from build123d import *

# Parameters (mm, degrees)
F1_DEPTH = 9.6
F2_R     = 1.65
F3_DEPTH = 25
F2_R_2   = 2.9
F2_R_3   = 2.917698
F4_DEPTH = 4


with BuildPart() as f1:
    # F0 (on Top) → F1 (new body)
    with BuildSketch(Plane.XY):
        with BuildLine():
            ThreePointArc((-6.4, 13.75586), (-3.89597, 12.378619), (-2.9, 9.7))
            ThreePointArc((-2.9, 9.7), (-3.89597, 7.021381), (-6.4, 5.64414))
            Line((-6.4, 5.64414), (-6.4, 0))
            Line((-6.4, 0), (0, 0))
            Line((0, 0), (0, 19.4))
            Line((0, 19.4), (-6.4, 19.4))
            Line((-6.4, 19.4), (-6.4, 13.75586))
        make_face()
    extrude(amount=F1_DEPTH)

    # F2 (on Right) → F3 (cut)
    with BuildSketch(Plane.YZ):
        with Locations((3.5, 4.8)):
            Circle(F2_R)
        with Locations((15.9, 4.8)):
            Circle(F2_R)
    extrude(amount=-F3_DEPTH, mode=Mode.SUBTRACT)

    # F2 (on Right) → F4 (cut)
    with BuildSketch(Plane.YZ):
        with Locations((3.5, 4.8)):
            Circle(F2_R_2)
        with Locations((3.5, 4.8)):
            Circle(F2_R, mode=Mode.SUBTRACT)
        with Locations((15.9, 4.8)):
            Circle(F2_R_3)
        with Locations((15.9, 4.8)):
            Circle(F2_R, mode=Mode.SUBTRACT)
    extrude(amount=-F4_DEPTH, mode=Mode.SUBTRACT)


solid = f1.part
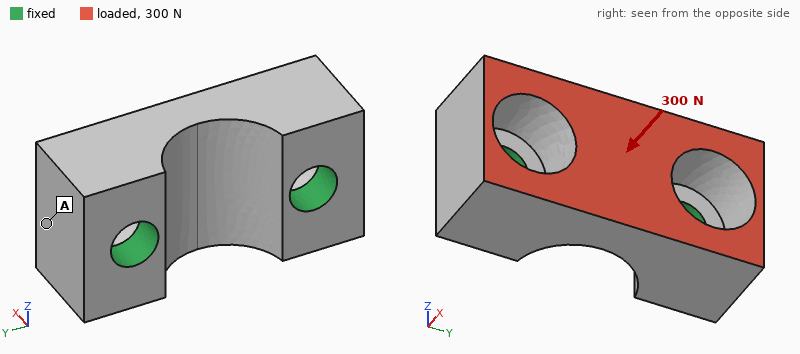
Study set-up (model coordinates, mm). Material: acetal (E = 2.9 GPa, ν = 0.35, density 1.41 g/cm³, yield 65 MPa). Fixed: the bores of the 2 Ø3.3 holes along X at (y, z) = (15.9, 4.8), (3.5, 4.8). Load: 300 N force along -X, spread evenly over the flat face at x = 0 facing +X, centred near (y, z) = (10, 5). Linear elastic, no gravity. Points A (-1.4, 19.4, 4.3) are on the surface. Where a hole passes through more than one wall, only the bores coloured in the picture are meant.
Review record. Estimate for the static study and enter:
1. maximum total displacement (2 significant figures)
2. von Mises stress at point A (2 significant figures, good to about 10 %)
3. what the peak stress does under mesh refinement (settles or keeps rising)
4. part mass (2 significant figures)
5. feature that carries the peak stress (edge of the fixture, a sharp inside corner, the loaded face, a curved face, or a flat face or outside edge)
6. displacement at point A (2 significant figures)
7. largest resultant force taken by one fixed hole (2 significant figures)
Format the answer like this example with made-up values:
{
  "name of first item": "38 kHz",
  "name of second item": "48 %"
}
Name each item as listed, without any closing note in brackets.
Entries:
{
  "maximum total displacement": "27 µm",
  "von Mises stress at point A": "4.2 MPa",
  "what the peak stress does under mesh refinement": "keeps rising",
  "part mass": "1.0 g",
  "feature that carries the peak stress": "a sharp inside corner",
  "displacement at point A": "8.4 µm",
  "largest resultant force taken by one fixed hole": "160 N"
}
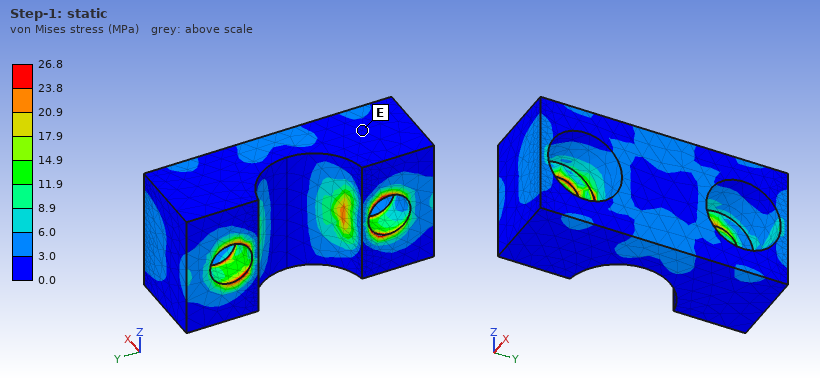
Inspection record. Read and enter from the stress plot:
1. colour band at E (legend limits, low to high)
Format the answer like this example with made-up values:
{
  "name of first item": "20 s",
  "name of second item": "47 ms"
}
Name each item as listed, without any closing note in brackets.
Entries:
{
  "colour band at E": "0.0 to 3.0 MPa"
}
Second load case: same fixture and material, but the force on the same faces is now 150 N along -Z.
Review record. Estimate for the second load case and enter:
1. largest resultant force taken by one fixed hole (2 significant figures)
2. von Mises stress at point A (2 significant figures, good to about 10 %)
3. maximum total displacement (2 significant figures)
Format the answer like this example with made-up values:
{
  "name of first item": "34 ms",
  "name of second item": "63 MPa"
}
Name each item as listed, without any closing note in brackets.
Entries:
{
  "largest resultant force taken by one fixed hole": "75 N",
  "von Mises stress at point A": "11 MPa",
  "maximum total displacement": "82 µm"
}
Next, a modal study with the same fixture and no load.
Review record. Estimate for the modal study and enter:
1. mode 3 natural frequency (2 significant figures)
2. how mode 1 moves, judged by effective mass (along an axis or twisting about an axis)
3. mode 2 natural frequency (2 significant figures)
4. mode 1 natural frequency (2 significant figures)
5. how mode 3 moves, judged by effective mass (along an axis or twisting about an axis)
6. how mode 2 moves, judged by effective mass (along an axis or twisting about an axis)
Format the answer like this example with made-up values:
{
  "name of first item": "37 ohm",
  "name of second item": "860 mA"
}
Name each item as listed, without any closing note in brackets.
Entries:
{
  "mode 3 natural frequency": "19 kHz",
  "how mode 1 moves, judged by effective mass": "along Z",
  "mode 2 natural frequency": "17 kHz",
  "mode 1 natural frequency": "11 kHz",
  "how mode 3 moves, judged by effective mass": "along Y",
  "how mode 2 moves, judged by effective mass": "twisting about X"
}
